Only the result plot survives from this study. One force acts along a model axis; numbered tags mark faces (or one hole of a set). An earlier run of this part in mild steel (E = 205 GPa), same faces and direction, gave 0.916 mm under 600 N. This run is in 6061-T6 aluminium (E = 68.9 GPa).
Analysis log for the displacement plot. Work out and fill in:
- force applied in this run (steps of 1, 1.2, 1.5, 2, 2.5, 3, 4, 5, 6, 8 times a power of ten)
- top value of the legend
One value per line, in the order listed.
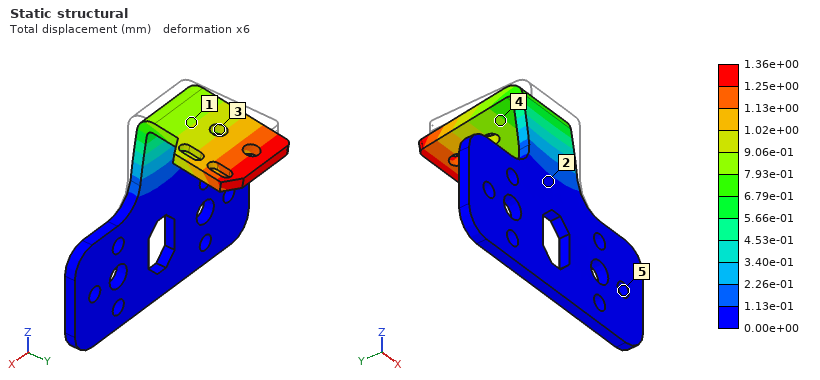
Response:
300 N
1.36e+00 mm
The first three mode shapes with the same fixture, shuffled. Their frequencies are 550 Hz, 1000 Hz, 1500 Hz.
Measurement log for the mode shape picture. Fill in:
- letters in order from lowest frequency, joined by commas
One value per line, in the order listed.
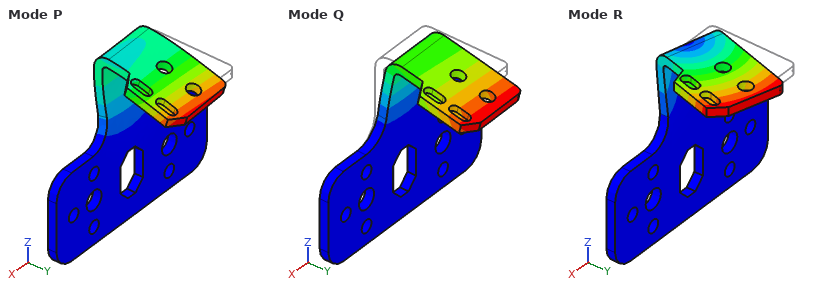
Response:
Q, R, P
